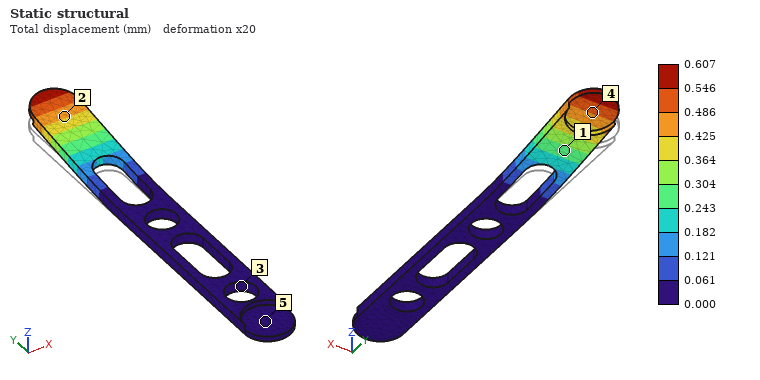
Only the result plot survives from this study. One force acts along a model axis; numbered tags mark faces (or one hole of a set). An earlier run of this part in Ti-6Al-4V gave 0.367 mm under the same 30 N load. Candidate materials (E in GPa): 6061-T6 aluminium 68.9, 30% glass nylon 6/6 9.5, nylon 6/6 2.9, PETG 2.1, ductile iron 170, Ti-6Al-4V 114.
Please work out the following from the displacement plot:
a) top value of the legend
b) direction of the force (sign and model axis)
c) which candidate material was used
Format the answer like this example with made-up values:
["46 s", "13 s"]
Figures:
["0.607 mm", "+Z", "6061-T6 aluminium"]
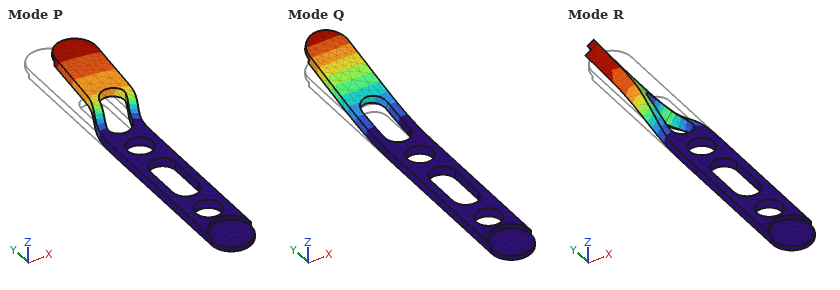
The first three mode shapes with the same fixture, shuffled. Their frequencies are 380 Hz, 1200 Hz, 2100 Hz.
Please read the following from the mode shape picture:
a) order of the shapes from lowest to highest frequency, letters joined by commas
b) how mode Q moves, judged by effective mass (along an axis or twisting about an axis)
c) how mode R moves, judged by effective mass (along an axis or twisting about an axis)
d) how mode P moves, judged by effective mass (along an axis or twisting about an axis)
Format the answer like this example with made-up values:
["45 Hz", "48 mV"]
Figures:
["Q, P, R", "along Z", "twisting about Y", "along X"]
